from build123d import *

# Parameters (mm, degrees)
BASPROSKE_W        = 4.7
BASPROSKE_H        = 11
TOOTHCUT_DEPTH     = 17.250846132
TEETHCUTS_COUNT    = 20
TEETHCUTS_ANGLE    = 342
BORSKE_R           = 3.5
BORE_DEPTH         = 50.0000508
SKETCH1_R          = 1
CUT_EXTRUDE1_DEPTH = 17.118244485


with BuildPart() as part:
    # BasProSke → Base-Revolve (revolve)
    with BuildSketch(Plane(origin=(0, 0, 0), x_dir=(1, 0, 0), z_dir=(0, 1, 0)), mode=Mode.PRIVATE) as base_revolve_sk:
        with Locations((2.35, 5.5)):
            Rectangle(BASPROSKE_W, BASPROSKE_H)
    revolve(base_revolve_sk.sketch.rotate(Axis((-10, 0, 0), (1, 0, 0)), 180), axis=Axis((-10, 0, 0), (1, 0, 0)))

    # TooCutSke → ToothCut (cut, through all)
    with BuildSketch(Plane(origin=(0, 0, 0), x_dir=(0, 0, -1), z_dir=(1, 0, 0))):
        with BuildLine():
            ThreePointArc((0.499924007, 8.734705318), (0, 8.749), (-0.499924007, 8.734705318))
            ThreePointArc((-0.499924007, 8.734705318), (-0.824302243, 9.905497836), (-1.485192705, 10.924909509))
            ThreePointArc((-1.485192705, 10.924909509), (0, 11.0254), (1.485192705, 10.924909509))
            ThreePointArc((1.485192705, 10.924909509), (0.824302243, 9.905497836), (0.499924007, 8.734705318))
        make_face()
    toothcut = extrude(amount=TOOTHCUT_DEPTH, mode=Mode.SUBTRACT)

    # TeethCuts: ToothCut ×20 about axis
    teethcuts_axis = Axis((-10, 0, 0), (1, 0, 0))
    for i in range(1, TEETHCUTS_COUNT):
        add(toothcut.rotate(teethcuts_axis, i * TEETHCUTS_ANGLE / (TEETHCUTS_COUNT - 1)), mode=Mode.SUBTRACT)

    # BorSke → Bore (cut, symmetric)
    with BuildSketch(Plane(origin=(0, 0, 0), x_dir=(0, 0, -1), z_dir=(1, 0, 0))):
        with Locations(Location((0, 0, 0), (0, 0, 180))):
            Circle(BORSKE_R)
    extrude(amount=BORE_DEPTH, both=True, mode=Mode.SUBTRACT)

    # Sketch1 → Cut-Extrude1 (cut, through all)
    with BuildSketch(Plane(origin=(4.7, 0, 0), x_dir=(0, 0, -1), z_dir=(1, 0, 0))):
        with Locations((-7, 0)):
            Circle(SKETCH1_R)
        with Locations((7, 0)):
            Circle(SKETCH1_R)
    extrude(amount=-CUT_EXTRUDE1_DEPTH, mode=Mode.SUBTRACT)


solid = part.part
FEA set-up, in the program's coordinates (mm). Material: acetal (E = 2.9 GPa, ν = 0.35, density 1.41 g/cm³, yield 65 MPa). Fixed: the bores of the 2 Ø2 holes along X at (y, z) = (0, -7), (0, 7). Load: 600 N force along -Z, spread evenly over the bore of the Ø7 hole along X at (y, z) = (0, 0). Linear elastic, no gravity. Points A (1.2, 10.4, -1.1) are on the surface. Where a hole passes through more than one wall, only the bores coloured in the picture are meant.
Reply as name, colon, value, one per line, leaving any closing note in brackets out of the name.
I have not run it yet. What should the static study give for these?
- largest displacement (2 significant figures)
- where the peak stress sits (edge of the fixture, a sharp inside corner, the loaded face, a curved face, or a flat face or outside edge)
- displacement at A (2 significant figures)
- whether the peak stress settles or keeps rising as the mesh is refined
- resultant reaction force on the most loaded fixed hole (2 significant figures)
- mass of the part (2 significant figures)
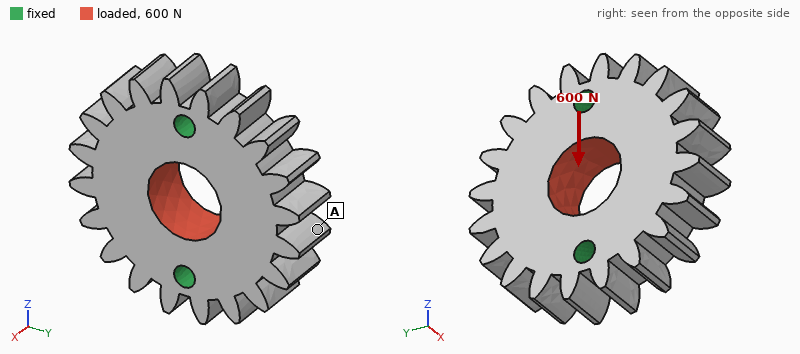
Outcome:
largest displacement: 28 µm
where the peak stress sits: edge of the fixture
displacement at A: 13 µm
whether the peak stress settles or keeps rising as the mesh is refined: keeps rising
resultant reaction force on the most loaded fixed hole: 300 N
mass of the part: 1.7 g
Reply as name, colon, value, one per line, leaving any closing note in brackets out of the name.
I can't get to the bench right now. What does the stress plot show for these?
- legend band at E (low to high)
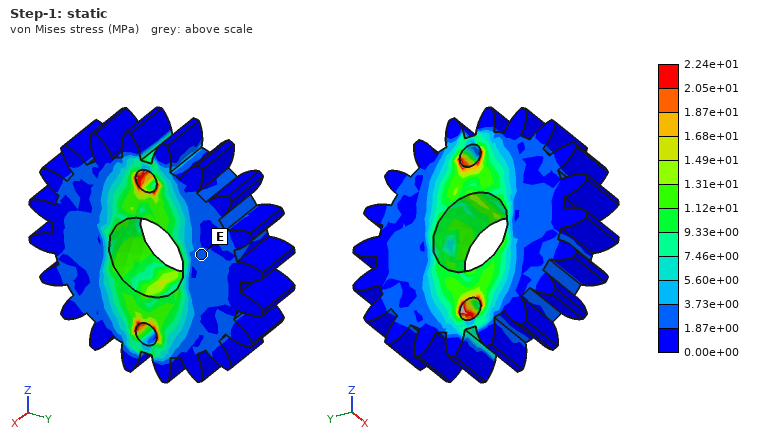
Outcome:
legend band at E: 1.87e+00 to 3.73e+00 MPa
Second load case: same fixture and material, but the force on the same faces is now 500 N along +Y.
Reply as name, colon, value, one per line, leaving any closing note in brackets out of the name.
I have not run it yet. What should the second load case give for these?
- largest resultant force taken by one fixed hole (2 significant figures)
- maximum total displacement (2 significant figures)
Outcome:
largest resultant force taken by one fixed hole: 250 N
maximum total displacement: 26 µm
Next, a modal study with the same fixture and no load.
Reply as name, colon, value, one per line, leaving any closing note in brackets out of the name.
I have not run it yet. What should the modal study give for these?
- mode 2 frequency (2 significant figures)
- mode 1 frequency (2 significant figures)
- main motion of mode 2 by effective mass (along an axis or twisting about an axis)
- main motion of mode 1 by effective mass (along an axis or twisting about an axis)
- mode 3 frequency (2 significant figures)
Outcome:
mode 2 frequency: 9500 Hz
mode 1 frequency: 8400 Hz
main motion of mode 2 by effective mass: along X
main motion of mode 1 by effective mass: twisting about Z
mode 3 frequency: 17 kHz
